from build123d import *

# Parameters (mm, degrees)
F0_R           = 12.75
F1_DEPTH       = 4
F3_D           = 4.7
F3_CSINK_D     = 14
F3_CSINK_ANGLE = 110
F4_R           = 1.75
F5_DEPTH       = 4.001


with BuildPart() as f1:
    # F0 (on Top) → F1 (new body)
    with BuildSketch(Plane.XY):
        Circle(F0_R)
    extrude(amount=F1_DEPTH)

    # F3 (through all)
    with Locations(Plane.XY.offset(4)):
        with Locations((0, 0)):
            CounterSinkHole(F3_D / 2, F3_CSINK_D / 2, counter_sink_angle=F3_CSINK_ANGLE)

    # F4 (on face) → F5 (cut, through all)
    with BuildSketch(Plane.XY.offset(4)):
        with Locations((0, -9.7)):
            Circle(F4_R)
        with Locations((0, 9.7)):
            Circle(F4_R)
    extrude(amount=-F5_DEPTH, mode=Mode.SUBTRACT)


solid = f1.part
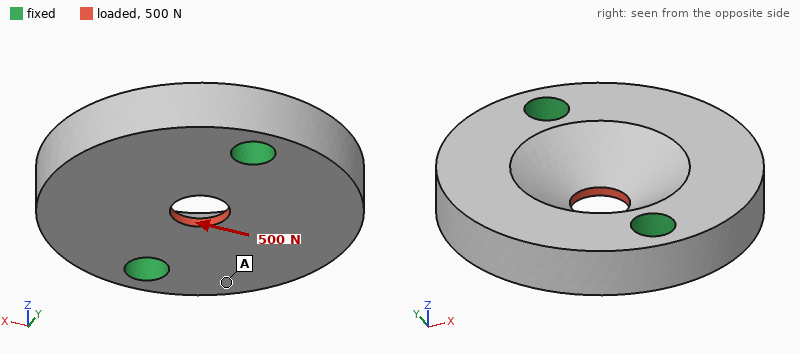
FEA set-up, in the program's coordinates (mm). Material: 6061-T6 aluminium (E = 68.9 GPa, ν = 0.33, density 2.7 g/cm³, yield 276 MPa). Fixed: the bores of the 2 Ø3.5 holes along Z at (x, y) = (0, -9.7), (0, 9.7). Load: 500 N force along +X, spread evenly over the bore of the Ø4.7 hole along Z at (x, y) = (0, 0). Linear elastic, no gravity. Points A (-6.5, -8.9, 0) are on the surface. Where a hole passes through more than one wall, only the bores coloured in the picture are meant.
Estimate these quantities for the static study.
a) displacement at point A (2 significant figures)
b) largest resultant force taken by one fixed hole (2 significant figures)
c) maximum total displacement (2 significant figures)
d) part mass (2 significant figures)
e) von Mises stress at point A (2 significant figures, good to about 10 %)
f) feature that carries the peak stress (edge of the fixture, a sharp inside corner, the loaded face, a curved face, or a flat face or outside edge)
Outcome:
1.3 µm
250 N
4.0 µm
4.6 g
7.3 MPa
the loaded face
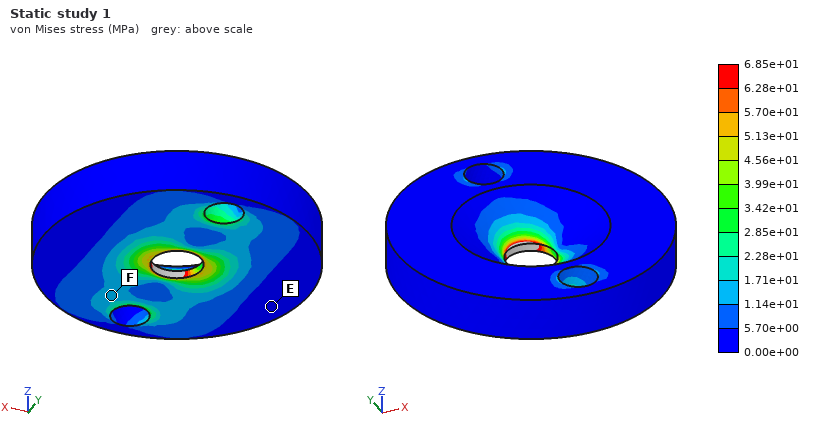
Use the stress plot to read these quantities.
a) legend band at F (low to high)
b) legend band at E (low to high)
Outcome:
1.14e+01 to 1.71e+01 MPa
0.00e+00 to 5.70e+00 MPa
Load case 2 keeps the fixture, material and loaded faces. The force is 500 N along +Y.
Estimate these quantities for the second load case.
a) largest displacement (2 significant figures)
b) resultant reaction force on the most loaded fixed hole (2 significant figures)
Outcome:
3.1 µm
250 N
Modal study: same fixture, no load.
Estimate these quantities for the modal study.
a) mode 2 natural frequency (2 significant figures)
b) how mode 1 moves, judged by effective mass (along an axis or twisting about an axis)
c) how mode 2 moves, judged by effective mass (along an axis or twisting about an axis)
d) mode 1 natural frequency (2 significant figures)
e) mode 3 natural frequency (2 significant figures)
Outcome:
21 kHz
twisting about Y
along Z
19 kHz
46 kHz
